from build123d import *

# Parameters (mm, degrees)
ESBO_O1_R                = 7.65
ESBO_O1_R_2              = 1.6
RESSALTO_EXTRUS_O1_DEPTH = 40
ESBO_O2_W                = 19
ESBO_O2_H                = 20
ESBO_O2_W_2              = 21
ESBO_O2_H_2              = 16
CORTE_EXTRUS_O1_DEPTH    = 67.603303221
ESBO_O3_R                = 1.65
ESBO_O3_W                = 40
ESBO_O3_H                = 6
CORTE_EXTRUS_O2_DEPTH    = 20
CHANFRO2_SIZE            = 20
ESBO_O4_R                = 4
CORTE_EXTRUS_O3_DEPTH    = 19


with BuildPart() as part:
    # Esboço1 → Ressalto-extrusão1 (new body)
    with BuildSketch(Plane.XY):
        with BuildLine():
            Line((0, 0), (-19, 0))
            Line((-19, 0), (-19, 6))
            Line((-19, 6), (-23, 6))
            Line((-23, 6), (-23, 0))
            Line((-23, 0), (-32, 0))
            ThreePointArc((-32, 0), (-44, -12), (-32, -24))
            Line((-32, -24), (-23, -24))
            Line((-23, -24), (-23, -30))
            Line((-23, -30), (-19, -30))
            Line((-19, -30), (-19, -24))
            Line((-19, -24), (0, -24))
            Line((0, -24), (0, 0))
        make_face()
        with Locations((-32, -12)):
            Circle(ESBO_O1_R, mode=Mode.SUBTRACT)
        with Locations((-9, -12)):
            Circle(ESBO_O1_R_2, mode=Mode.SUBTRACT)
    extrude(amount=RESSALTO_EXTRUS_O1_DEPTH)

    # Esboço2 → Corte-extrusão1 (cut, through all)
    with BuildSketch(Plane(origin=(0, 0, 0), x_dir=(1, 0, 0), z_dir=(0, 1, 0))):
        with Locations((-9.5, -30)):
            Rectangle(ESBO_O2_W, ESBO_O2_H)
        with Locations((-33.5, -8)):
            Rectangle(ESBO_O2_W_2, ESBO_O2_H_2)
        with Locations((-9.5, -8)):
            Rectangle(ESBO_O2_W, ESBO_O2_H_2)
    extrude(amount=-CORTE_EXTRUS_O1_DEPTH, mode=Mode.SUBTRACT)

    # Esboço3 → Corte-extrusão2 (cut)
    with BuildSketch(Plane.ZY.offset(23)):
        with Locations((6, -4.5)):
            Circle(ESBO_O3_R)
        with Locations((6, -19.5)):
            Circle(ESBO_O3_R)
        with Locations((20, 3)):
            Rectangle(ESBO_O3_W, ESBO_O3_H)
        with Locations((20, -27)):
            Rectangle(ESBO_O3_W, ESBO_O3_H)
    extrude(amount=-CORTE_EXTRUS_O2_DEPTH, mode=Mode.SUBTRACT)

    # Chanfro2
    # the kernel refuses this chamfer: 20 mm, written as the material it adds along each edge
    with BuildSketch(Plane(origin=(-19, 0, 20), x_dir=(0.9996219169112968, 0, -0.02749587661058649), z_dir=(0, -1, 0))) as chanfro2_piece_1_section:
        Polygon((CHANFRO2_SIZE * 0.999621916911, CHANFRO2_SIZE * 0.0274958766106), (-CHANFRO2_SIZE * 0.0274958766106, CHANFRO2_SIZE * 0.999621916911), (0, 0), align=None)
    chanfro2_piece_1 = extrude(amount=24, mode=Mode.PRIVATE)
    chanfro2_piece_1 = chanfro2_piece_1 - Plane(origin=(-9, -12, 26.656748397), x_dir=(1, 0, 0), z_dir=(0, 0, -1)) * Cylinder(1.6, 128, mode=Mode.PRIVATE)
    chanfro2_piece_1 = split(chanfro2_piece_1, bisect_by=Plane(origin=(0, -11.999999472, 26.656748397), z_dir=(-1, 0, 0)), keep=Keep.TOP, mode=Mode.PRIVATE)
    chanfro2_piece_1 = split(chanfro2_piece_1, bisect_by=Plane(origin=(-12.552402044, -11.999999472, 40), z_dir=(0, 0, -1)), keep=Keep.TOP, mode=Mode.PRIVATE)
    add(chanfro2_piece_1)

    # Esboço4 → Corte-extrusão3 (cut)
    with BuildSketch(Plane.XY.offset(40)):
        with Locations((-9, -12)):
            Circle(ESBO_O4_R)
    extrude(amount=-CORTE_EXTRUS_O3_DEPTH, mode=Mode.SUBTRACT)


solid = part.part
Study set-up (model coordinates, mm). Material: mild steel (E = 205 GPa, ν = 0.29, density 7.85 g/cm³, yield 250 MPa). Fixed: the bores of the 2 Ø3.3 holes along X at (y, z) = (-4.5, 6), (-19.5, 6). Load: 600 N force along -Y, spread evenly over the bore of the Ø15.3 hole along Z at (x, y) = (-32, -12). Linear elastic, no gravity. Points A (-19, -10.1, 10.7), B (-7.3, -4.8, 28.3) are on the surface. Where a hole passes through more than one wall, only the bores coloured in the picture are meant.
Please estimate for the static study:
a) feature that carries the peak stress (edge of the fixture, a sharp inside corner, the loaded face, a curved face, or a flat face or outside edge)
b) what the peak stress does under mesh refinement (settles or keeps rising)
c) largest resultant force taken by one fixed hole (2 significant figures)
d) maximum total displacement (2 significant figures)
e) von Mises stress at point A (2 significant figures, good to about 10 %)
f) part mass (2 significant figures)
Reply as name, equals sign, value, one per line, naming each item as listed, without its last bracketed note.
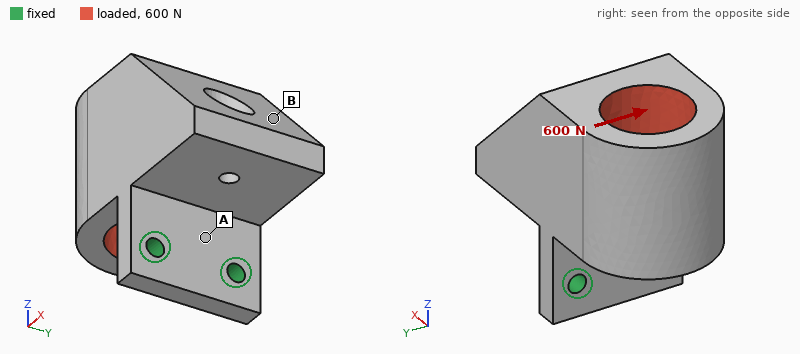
feature that carries the peak stress = edge of the fixture
what the peak stress does under mesh refinement = keeps rising
largest resultant force taken by one fixed hole = 910 N
maximum total displacement = 20 µm
von Mises stress at point A = 15 MPa
part mass = 130 g
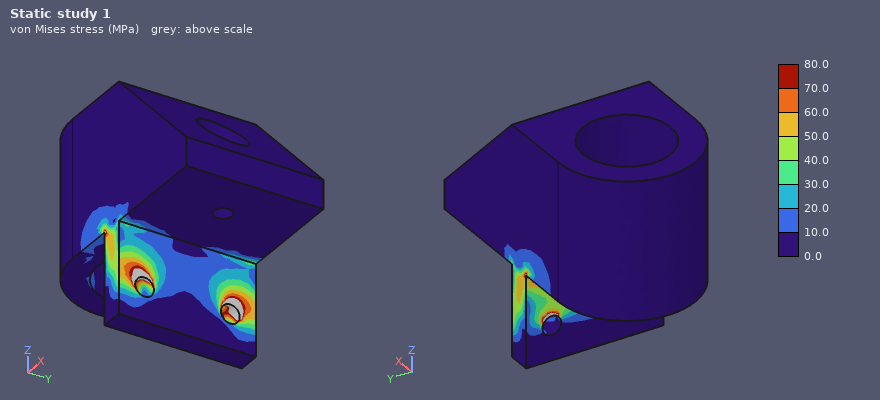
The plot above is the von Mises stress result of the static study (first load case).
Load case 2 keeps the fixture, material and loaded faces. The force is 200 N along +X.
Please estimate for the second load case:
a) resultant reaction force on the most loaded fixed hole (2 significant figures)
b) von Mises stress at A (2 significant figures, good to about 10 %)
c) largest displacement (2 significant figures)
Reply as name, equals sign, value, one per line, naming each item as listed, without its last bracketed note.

resultant reaction force on the most loaded fixed hole = 100 N
von Mises stress at A = 42 MPa
largest displacement = 50 µm
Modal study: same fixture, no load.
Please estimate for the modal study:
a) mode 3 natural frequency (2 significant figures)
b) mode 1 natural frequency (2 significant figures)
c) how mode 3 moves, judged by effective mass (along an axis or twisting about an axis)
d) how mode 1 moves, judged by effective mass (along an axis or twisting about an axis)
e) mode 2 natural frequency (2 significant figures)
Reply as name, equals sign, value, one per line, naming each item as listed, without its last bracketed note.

mode 3 natural frequency = 6000 Hz
mode 1 natural frequency = 1200 Hz
how mode 3 moves, judged by effective mass = along Y
how mode 1 moves, judged by effective mass = along X
mode 2 natural frequency = 3600 Hz
